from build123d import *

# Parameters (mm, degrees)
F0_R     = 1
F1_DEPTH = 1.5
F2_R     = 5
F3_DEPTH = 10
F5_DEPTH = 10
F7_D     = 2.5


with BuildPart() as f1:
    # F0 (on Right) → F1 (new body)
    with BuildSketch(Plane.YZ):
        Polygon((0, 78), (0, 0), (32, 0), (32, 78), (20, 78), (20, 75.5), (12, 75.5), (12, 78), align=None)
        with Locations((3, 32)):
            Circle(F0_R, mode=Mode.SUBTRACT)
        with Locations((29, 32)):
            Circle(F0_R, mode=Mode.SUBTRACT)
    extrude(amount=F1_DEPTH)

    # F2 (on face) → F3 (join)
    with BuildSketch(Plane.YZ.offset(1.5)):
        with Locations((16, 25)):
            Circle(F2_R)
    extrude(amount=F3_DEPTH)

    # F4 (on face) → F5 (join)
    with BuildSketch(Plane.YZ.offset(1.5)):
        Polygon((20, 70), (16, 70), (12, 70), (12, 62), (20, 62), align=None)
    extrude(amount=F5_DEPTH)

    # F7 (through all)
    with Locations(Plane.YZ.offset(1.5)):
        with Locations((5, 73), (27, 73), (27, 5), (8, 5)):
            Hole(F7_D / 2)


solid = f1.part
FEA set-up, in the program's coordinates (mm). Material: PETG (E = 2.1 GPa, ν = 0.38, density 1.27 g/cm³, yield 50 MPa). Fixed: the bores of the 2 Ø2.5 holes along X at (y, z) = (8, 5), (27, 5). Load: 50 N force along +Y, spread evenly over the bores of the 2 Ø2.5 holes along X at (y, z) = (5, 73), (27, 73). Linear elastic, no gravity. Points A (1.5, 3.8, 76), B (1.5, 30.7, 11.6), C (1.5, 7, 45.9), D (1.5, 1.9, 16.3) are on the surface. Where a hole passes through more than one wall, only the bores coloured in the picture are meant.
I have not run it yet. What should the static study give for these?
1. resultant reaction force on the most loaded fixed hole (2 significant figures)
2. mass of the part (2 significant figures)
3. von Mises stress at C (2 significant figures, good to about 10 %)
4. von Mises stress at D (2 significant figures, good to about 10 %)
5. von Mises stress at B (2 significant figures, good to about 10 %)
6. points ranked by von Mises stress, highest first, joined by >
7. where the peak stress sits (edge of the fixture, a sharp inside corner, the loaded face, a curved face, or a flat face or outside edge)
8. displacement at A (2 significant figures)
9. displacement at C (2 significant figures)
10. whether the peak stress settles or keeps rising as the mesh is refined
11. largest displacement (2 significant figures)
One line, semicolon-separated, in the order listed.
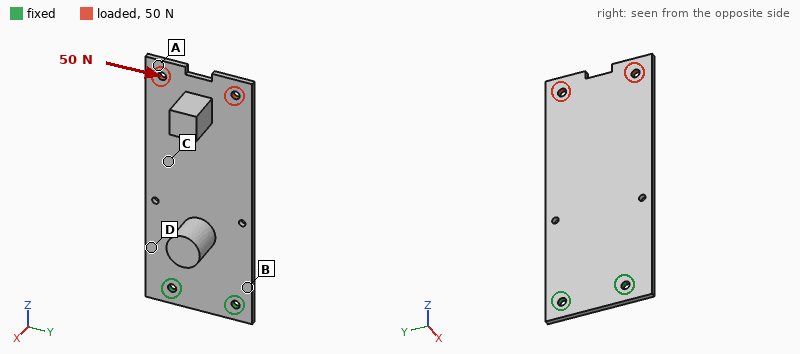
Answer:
170 N; 6.5 g; 3.5 MPa; 8.2 MPa; 11 MPa; B > D > C > A; edge of the fixture; 0.95 mm; 0.44 mm; keeps rising; 1.00 mm
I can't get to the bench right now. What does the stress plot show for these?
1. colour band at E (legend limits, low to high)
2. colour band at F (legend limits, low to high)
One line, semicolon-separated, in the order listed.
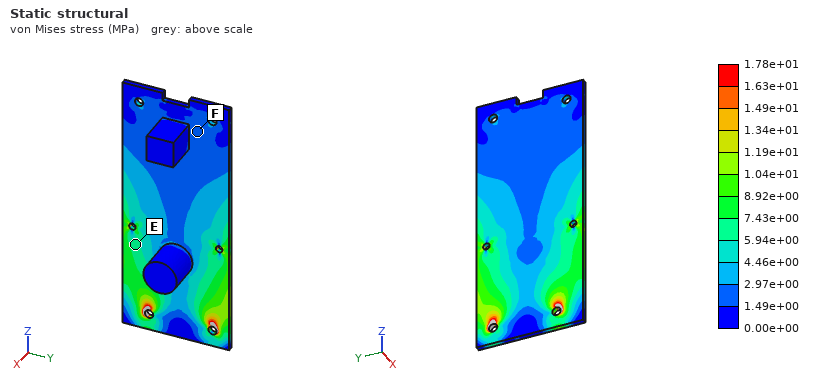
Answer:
5.94e+00 to 7.43e+00 MPa; 1.49e+00 to 2.97e+00 MPa
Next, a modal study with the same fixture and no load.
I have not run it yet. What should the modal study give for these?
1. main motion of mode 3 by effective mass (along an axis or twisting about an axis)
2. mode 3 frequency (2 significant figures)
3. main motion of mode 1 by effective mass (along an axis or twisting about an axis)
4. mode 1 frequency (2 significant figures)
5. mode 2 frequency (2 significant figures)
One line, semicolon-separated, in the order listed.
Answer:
along X; 320 Hz; along X; 53 Hz; 280 Hz
